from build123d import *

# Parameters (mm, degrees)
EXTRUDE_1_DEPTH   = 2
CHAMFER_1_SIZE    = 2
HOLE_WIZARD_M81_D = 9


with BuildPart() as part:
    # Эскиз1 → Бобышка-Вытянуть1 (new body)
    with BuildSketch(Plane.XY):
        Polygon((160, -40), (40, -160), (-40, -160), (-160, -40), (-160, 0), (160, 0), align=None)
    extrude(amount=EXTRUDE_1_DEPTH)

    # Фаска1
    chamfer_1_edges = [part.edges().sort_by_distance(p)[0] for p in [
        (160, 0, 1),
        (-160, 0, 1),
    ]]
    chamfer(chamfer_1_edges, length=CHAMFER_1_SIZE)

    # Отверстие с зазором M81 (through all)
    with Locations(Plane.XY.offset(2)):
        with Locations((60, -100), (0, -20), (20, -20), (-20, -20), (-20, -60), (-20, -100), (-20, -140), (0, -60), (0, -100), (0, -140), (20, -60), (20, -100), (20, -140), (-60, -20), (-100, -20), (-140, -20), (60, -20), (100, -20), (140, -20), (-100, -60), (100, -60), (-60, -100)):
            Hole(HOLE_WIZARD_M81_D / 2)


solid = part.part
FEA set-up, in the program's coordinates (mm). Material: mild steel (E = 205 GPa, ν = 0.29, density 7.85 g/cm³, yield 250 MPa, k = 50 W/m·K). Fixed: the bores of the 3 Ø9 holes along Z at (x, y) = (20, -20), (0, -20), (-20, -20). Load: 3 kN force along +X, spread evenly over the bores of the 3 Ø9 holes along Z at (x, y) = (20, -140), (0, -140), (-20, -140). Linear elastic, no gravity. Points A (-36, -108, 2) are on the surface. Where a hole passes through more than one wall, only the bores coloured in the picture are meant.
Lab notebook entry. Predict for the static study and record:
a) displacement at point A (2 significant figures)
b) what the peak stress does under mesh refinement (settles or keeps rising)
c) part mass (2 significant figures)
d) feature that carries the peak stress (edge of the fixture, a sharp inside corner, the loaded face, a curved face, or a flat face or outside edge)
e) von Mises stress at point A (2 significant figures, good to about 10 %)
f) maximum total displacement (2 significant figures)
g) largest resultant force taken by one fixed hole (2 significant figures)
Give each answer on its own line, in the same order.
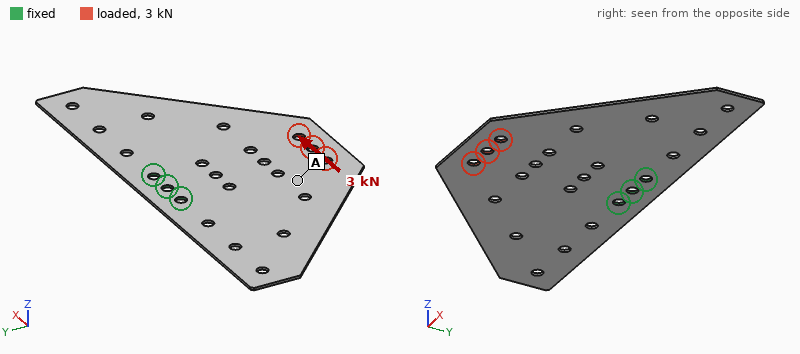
0.096 mm
keeps rising
560 g
edge of the fixture
20 MPa
0.16 mm
7.4 kN
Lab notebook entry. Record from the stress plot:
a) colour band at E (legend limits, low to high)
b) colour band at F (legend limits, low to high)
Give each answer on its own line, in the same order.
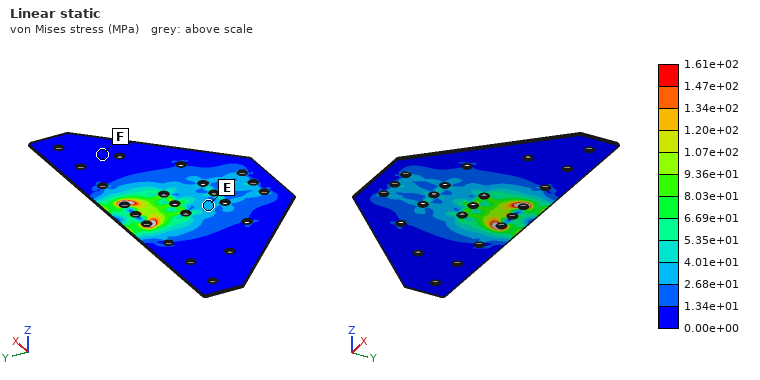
2.68e+01 to 4.01e+01 MPa
0.00e+00 to 1.34e+01 MPa
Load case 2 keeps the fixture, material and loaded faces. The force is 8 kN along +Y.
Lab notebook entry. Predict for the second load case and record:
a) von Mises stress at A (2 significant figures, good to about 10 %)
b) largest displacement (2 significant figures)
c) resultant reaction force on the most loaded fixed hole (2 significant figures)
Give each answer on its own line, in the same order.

35 MPa
35 µm
3.3 kN
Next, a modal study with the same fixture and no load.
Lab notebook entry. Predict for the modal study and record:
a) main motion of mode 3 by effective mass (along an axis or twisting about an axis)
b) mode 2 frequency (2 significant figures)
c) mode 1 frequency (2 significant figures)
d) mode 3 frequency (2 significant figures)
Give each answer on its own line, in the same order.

along Z
90 Hz
89 Hz
110 Hz
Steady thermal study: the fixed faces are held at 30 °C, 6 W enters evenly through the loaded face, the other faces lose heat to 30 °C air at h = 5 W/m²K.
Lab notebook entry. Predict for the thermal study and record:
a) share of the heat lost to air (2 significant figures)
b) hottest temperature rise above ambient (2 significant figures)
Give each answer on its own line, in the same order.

65 %
40 K
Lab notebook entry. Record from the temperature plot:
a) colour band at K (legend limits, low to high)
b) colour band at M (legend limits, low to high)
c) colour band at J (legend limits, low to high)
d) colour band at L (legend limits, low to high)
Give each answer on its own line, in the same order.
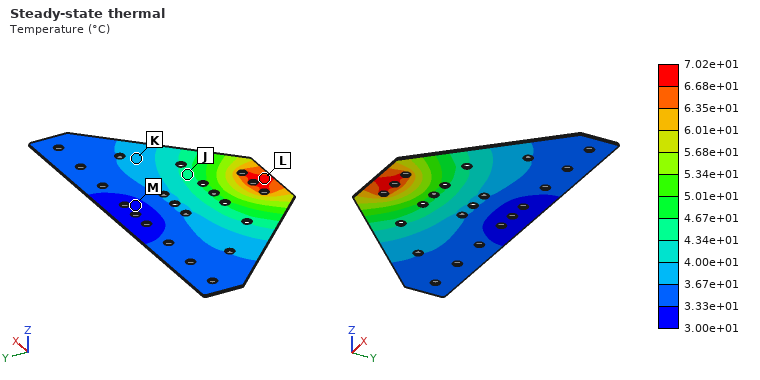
3.67e+01 to 4.00e+01 °C
3.00e+01 to 3.33e+01 °C
4.34e+01 to 4.67e+01 °C
6.68e+01 to 7.02e+01 °C
